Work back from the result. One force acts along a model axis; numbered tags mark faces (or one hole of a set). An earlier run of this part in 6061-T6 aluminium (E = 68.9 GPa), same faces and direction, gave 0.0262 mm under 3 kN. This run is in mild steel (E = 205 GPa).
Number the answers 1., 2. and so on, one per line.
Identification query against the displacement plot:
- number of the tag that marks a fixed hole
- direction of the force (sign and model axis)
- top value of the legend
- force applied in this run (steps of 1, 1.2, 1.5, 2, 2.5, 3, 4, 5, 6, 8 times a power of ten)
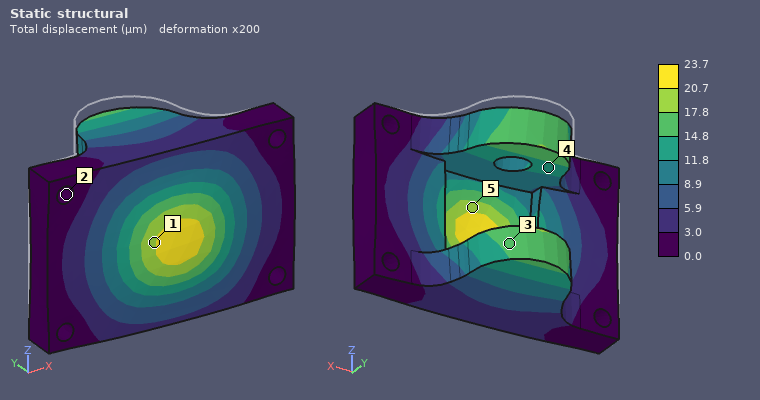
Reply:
1. 2
2. -Y
3. 23.7 µm
4. 8 kN
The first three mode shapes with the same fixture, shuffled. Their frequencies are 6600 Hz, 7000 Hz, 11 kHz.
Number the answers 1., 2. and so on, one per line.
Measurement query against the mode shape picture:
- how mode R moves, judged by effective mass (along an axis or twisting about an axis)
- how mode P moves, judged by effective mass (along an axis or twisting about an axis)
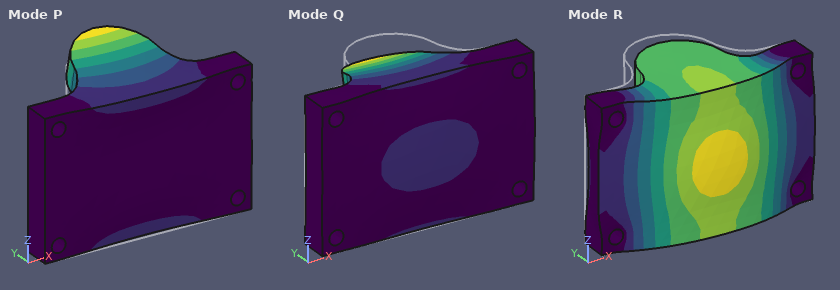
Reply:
1. along Y
2. along Z
